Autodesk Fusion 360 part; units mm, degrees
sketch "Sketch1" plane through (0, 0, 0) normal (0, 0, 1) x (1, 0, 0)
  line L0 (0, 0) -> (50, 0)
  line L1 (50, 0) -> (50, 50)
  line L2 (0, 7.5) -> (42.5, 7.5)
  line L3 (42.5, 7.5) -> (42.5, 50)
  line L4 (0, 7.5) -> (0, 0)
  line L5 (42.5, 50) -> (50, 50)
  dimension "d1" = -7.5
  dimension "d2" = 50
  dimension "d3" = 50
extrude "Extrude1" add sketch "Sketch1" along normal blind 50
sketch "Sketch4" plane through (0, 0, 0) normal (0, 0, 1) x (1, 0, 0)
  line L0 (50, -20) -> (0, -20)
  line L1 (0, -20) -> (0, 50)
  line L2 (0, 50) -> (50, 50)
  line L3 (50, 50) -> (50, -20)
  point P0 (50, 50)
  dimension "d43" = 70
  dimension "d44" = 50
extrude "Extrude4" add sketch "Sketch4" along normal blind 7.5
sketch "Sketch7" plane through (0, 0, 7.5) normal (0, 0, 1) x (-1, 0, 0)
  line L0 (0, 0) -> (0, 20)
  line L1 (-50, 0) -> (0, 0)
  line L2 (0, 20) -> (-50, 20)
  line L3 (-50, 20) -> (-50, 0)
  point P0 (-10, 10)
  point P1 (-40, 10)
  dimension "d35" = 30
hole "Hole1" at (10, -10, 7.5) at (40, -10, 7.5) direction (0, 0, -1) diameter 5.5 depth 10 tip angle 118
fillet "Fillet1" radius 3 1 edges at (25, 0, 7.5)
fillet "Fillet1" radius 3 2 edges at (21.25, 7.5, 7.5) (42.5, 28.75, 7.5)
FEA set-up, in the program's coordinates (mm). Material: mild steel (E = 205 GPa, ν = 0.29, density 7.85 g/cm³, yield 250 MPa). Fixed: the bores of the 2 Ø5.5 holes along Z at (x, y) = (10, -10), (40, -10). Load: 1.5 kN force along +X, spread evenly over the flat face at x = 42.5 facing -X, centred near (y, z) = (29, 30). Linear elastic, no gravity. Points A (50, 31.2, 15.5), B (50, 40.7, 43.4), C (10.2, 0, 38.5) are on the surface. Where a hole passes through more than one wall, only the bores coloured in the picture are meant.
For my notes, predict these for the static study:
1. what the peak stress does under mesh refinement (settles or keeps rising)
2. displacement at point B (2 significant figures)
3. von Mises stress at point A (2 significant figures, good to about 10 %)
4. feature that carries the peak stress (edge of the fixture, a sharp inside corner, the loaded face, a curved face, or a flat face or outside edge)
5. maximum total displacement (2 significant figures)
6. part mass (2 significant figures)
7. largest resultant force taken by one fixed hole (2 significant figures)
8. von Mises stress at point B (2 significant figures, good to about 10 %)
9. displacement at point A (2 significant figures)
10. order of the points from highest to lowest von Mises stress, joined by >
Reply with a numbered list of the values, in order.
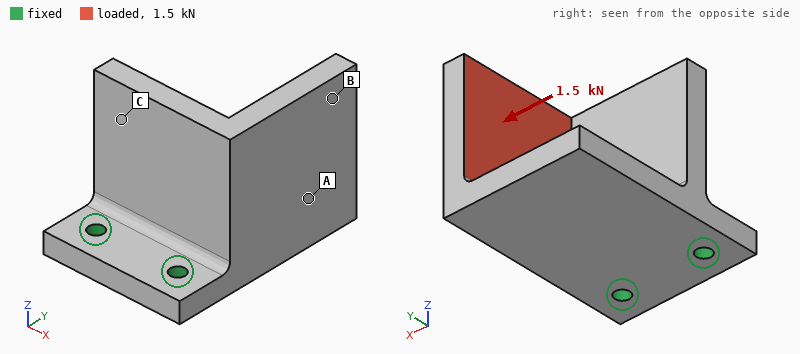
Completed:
1. keeps rising
2. 42 µm
3. 22 MPa
4. edge of the fixture
5. 55 µm
6. 440 g
7. 2.3 kN
8. 13 MPa
9. 15 µm
10. A > B > C
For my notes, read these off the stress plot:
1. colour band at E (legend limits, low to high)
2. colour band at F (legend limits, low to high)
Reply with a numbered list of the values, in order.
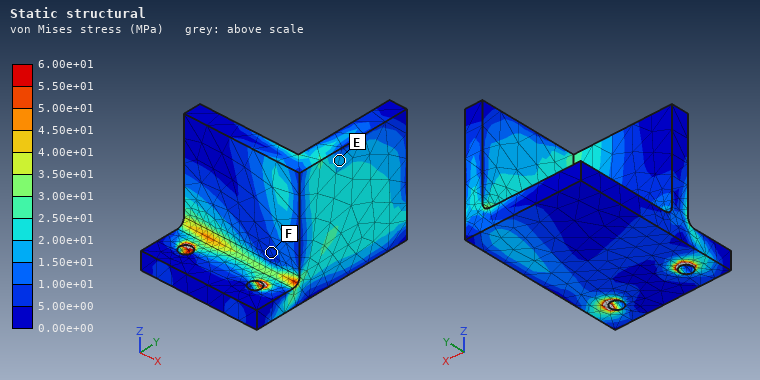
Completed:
1. 1.50e+01 to 2.00e+01 MPa
2. 5.00e+00 to 1.00e+01 MPa
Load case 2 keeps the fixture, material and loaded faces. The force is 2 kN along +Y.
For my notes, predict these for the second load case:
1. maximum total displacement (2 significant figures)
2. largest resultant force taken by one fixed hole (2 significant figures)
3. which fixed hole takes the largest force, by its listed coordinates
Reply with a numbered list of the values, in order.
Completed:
1. 0.17 mm
2. 2.1 kN
3. (40, -10)
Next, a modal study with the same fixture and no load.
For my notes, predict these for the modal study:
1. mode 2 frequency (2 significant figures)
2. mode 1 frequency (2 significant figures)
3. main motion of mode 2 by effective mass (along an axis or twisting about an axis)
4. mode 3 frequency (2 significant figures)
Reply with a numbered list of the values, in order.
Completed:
1. 3100 Hz
2. 1100 Hz
3. along X
4. 4400 Hz
